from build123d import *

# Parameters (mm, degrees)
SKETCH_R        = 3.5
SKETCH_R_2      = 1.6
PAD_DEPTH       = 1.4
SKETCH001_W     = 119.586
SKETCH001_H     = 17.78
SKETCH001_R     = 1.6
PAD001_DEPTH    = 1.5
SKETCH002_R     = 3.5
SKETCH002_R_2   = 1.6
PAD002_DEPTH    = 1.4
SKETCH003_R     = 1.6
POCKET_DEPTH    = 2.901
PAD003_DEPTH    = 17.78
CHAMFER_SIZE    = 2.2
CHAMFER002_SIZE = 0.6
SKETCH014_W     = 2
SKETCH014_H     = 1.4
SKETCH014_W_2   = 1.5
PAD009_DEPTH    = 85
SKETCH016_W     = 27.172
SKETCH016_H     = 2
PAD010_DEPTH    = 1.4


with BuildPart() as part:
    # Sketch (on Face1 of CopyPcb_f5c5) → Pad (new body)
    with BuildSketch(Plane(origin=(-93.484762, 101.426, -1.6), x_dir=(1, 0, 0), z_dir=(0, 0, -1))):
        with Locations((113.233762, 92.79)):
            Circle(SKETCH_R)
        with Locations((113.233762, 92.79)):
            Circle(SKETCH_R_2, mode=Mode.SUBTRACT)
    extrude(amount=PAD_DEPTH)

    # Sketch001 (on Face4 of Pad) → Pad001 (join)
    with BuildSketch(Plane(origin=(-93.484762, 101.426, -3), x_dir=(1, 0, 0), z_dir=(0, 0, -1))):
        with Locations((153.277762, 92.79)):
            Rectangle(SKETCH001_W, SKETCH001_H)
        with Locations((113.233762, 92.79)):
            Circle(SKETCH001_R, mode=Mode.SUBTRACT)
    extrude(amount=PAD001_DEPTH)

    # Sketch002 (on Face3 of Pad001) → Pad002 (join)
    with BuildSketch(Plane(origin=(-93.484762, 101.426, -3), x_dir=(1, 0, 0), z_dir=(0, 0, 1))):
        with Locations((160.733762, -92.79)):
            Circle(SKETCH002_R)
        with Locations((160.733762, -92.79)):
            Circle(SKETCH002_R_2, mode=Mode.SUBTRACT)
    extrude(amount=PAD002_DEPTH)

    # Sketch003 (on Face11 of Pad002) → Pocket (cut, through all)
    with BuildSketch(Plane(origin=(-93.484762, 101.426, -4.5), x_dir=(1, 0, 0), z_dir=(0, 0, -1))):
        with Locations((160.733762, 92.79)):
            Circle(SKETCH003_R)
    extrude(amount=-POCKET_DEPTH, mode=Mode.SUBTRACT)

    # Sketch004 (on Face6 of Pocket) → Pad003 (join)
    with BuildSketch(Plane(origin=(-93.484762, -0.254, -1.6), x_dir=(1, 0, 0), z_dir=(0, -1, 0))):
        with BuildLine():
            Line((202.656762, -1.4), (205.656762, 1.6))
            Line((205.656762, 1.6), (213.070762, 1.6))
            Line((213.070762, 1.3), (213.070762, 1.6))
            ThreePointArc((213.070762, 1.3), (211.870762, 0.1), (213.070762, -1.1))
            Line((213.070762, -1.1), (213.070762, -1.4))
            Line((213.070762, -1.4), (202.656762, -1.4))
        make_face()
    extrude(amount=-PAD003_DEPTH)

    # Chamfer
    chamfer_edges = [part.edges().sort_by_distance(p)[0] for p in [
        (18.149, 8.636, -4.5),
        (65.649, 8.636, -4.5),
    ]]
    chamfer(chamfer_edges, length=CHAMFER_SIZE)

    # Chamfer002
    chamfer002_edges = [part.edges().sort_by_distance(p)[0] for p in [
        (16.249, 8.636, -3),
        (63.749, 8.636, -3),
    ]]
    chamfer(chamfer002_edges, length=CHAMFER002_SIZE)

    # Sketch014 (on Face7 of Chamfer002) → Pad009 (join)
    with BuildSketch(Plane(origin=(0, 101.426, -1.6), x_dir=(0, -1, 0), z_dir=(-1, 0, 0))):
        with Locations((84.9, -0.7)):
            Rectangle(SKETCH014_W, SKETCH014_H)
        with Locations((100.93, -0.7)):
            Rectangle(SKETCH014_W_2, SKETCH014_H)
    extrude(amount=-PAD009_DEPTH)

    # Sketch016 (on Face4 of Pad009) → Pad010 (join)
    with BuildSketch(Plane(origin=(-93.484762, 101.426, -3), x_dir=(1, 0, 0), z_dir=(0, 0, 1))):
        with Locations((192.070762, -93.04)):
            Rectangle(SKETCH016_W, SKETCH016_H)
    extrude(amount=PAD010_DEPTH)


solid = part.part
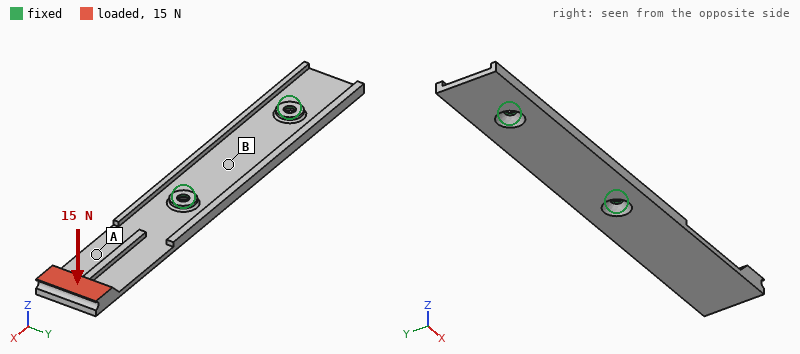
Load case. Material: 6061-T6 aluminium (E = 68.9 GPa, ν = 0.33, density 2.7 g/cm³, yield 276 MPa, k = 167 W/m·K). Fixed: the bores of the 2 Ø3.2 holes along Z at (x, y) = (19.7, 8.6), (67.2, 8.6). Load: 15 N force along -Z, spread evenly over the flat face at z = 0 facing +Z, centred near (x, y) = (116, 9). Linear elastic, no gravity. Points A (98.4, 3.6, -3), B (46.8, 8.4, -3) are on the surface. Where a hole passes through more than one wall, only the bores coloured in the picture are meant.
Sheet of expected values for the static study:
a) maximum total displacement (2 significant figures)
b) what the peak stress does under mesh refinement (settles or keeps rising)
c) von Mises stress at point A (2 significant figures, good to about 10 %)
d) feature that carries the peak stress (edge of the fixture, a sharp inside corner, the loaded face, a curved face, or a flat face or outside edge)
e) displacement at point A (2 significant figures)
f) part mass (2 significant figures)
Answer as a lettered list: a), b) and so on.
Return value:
a) 0.94 mm
b) keeps rising
c) 16 MPa
d) edge of the fixture
e) 0.41 mm
f) 11 g
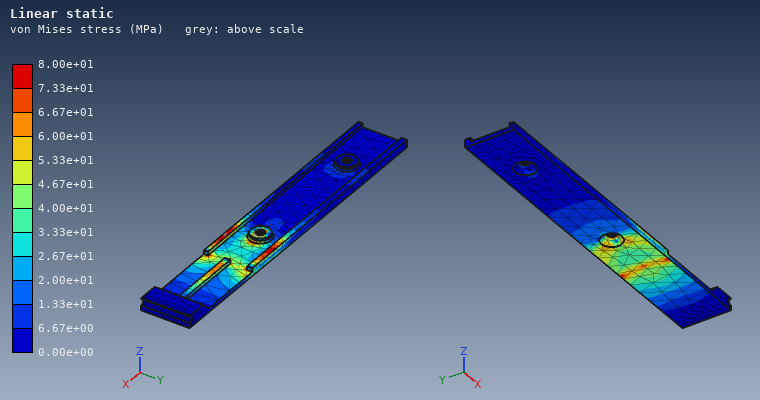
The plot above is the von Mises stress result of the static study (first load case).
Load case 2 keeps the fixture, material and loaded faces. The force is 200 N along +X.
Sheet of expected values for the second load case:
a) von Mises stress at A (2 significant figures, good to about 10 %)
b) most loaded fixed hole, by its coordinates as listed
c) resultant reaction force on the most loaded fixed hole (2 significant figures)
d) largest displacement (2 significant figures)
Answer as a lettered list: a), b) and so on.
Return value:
a) 47 MPa
b) (67.2, 8.6)
c) 210 N
d) 1.4 mm
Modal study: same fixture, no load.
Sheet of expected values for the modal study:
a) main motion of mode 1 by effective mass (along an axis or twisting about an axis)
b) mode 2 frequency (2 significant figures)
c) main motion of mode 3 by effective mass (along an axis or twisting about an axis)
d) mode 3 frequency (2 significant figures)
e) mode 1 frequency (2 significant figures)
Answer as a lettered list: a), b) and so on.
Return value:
a) along Z
b) 2100 Hz
c) along Y
d) 2900 Hz
e) 440 Hz
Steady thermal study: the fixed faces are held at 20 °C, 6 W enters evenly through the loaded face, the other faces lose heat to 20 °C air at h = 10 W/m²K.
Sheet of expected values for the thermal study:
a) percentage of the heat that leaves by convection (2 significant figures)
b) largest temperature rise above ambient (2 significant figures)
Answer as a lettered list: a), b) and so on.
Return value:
a) 12 %
b) 55 K
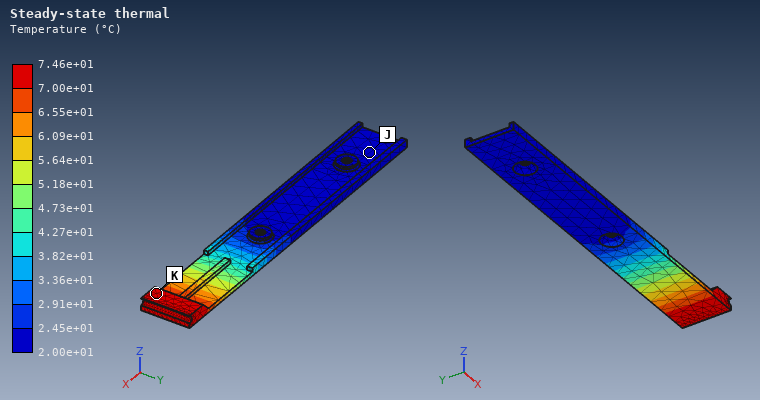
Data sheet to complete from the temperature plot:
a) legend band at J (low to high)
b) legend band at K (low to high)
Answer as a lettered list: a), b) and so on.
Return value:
a) 2.00e+01 to 2.45e+01 °C
b) 7.00e+01 to 7.46e+01 °C
